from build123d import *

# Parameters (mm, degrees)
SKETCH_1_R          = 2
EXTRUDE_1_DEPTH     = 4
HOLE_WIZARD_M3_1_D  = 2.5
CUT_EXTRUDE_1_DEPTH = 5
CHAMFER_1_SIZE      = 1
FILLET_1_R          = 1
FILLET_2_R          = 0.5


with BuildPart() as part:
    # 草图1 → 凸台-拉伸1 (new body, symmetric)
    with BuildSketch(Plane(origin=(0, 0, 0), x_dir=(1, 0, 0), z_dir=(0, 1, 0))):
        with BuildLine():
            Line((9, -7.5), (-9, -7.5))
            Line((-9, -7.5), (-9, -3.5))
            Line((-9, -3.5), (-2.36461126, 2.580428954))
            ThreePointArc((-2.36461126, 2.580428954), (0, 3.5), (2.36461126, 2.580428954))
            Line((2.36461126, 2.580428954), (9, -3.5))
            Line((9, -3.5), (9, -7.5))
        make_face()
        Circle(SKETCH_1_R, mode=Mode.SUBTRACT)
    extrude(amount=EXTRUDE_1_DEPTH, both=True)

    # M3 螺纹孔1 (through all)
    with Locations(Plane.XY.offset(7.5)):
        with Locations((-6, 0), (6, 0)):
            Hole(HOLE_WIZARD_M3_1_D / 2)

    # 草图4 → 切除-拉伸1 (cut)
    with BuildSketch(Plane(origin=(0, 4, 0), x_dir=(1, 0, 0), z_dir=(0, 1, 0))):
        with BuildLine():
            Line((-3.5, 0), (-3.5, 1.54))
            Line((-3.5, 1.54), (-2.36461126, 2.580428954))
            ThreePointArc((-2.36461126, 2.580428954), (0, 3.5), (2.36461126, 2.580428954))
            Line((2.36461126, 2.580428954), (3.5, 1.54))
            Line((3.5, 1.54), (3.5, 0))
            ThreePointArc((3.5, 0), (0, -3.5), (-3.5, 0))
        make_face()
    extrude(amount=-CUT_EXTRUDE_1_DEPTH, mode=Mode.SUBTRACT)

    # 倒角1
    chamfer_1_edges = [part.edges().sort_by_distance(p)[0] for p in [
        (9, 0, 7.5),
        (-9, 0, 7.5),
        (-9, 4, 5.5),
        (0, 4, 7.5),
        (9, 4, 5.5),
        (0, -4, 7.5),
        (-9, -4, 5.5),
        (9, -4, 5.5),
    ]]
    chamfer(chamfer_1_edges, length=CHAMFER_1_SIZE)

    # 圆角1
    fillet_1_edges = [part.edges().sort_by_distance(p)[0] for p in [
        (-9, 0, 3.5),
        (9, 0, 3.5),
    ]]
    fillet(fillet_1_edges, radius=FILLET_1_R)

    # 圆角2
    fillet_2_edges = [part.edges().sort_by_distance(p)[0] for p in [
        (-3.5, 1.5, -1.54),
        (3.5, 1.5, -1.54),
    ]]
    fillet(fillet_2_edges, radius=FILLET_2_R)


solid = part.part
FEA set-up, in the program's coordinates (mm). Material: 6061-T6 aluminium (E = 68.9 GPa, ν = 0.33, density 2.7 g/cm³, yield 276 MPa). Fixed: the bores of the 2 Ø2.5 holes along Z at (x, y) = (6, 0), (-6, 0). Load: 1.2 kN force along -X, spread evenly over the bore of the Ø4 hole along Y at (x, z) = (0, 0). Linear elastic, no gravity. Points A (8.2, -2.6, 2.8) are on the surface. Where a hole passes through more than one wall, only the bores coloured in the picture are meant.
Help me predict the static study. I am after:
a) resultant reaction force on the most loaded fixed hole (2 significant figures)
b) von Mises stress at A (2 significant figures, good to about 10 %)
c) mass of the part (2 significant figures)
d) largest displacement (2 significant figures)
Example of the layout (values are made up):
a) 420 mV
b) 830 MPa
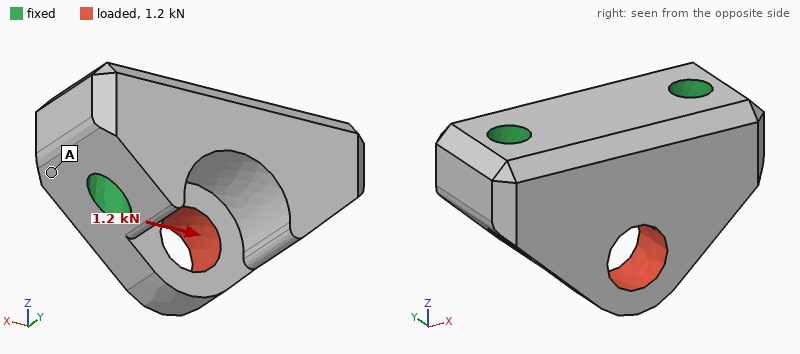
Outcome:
a) 660 N
b) 17 MPa
c) 2.2 g
d) 11 µm
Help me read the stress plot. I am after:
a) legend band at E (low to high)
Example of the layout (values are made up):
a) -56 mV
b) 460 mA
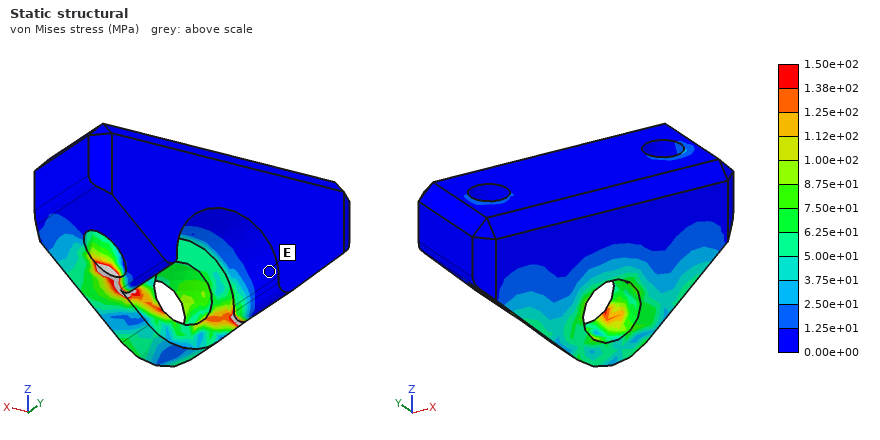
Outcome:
a) 0.00e+00 to 1.25e+01 MPa
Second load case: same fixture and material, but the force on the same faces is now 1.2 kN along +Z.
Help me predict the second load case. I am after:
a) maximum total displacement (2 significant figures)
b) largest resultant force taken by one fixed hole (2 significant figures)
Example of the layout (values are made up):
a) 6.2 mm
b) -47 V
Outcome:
a) 9.7 µm
b) 610 N
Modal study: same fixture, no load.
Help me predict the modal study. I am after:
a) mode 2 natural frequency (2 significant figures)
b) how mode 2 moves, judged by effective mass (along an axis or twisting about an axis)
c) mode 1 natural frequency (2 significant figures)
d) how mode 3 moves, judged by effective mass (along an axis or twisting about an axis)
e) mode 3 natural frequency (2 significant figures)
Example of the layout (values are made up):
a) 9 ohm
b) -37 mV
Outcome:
a) 110 kHz
b) along Y
c) 79 kHz
d) along Z
e) 120 kHz
